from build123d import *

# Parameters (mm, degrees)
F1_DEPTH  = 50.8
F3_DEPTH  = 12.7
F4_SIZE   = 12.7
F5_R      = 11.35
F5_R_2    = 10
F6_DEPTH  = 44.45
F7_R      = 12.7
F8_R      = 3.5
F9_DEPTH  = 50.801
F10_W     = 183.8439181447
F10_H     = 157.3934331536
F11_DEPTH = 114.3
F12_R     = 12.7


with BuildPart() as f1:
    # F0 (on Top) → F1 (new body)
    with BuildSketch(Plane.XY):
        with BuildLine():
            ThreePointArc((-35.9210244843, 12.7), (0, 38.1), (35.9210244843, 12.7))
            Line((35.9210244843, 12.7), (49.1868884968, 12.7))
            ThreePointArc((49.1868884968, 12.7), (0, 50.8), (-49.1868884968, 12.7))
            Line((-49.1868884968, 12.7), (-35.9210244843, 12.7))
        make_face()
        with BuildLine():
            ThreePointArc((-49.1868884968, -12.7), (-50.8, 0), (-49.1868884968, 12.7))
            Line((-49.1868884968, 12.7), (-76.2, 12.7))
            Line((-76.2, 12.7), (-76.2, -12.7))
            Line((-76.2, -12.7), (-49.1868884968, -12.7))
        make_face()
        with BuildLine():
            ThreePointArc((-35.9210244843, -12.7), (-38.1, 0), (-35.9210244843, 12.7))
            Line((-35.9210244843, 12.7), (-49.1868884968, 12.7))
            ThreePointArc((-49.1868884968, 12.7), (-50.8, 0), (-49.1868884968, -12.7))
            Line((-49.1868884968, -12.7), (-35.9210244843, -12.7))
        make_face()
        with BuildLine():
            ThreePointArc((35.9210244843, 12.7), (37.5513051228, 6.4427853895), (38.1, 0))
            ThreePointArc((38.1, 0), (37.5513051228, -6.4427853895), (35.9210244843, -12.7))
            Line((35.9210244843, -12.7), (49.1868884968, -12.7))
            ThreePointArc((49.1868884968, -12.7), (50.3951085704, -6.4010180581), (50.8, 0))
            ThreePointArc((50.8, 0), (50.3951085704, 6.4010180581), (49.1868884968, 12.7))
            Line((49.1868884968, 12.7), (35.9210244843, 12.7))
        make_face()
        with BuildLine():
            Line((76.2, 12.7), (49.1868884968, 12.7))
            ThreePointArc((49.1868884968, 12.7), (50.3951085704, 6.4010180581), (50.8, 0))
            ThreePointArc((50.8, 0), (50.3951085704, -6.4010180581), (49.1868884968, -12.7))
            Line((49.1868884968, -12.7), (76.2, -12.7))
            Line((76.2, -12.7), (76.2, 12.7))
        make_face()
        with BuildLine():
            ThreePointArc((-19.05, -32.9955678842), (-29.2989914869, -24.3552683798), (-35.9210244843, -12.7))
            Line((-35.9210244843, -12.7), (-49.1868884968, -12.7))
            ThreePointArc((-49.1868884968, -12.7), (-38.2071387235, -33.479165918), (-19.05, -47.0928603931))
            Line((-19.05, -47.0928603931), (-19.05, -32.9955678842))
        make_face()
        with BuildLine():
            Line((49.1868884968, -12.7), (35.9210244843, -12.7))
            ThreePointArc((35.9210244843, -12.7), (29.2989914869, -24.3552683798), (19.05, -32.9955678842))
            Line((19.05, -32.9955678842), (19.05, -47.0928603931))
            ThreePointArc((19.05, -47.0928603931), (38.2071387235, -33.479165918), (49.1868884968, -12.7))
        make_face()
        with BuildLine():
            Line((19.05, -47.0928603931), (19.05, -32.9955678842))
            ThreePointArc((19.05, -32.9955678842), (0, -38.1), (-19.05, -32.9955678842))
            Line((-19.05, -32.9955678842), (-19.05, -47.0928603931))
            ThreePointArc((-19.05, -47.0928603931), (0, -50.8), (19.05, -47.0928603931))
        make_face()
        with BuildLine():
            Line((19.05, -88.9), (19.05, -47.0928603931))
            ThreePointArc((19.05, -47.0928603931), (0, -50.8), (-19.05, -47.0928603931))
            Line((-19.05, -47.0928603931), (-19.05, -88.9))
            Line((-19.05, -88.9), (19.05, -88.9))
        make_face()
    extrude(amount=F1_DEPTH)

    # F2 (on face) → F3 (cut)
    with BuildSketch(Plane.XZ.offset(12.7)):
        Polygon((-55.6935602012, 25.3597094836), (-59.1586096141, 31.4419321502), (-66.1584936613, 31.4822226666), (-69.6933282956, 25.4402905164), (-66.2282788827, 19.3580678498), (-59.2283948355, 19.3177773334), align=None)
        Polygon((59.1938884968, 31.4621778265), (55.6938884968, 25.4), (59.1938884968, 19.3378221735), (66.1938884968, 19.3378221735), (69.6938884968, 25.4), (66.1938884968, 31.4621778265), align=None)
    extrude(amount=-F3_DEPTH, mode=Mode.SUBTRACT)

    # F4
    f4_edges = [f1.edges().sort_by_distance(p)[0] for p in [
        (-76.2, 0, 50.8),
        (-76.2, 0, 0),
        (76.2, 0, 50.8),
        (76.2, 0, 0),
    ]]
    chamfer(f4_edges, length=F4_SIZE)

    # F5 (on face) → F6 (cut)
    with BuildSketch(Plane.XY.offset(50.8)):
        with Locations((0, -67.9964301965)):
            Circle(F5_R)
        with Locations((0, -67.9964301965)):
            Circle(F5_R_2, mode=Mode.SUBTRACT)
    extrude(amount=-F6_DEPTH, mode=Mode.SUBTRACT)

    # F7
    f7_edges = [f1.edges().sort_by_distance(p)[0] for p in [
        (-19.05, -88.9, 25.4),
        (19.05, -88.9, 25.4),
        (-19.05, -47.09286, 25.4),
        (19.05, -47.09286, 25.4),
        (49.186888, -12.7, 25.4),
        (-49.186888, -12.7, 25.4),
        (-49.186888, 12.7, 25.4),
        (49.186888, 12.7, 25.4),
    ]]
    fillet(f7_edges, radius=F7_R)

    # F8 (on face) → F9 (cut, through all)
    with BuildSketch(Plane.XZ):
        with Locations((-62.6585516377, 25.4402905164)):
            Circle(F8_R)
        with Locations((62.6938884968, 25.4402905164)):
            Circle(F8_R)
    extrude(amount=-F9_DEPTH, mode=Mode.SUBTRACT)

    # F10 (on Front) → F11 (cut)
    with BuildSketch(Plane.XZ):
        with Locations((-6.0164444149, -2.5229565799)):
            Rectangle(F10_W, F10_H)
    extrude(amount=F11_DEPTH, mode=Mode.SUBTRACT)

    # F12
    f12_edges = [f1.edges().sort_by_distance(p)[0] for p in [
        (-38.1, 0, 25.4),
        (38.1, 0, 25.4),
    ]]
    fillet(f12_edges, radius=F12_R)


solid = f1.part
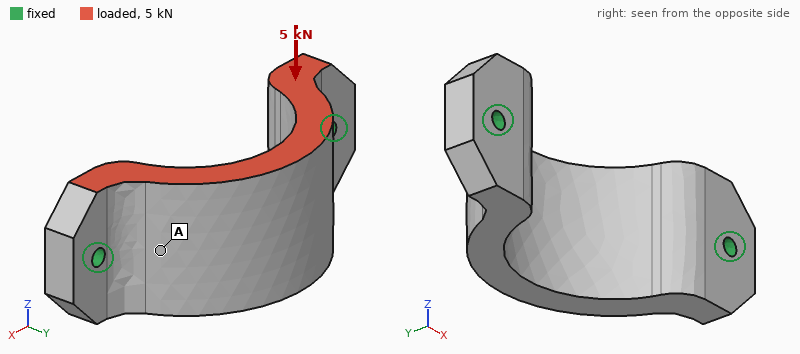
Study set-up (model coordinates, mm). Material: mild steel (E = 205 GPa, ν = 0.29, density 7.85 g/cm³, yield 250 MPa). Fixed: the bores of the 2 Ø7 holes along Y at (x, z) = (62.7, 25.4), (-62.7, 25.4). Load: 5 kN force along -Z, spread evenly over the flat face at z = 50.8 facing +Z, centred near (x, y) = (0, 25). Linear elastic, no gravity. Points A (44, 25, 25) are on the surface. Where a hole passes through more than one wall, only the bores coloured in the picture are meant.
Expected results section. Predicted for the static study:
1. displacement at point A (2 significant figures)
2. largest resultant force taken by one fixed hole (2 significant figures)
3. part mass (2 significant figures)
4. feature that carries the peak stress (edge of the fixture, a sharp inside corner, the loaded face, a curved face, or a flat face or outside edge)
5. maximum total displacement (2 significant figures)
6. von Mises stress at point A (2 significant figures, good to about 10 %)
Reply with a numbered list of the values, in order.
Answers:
1. 14 µm
2. 2.5 kN
3. 920 g
4. edge of the fixture
5. 36 µm
6. 19 MPa
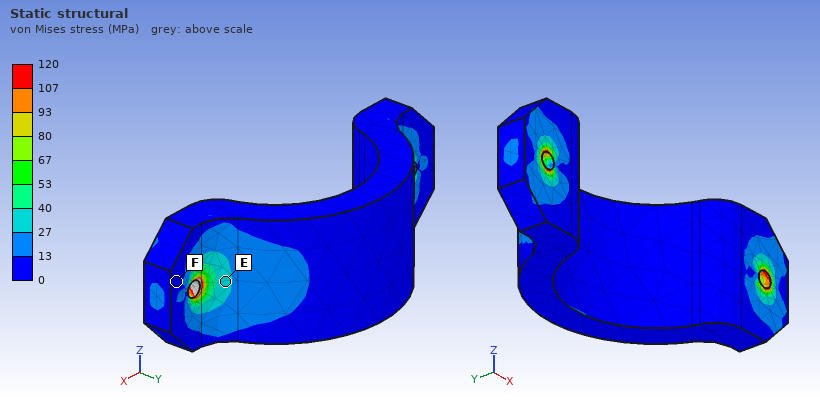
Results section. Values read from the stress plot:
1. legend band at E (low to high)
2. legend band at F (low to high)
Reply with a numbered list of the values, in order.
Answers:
1. 27 to 40 MPa
2. 0 to 13 MPa
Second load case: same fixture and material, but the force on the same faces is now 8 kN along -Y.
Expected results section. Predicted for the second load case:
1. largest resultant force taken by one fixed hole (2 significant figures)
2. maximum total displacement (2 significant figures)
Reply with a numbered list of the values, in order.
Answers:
1. 4.6 kN
2. 57 µm
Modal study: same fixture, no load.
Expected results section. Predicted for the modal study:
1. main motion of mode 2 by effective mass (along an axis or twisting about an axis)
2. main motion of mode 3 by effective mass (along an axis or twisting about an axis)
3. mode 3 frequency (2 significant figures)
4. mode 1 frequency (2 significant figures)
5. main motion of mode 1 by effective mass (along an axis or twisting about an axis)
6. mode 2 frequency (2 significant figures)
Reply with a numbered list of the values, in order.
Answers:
1. along X
2. along Y
3. 6800 Hz
4. 2400 Hz
5. along Z
6. 5700 Hz
